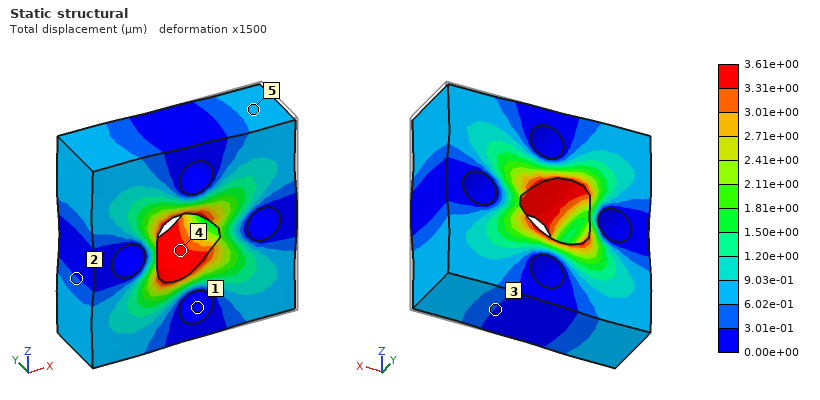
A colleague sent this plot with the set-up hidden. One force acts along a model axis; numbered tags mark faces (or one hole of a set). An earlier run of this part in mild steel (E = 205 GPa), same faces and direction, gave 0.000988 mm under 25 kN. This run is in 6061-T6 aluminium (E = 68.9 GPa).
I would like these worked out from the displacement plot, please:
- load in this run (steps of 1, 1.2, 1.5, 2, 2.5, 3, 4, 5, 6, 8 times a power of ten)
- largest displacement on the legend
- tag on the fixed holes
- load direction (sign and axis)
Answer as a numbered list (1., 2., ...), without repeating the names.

1. 30 kN
2. 3.61e+00 µm
3. 1
4. -X
